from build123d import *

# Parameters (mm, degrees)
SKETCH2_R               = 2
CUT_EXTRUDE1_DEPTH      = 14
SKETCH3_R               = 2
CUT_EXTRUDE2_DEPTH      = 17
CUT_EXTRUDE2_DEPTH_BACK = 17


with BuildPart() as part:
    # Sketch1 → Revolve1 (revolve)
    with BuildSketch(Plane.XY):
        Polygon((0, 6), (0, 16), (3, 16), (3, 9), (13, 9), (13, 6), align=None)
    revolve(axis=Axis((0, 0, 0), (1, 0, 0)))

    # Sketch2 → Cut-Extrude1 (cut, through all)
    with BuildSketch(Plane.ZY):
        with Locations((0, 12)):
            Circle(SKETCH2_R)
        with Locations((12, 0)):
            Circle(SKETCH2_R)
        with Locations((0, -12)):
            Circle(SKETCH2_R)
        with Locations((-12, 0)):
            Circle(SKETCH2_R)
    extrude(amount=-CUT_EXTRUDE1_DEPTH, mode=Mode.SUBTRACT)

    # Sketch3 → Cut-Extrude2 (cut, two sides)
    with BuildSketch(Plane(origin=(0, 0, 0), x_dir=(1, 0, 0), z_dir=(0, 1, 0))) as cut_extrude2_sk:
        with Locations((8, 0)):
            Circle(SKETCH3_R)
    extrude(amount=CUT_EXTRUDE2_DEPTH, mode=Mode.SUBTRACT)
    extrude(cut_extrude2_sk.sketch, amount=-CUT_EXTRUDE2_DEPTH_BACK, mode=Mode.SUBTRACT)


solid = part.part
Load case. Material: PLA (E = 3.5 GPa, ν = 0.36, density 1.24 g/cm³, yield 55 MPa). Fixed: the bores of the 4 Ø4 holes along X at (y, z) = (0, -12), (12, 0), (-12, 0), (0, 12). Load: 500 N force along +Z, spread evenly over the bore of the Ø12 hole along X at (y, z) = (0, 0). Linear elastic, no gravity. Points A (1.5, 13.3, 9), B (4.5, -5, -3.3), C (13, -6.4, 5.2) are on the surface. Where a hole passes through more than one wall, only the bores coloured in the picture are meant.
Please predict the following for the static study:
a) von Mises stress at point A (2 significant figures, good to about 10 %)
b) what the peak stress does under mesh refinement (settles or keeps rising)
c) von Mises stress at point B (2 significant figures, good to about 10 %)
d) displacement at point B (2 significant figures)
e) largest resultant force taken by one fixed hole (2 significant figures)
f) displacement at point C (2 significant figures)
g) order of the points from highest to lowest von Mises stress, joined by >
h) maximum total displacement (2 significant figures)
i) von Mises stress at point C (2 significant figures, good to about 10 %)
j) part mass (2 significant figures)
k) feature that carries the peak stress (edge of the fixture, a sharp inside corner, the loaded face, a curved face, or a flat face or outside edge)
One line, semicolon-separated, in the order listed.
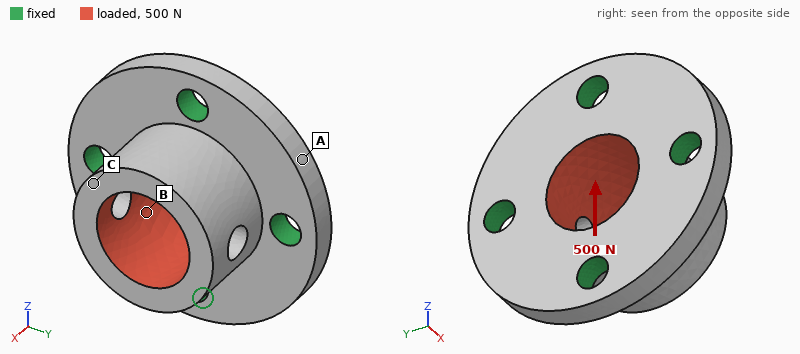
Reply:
1.5 MPa; keeps rising; 5.2 MPa; 17 µm; 180 N; 51 µm; B > C > A; 58 µm; 2.9 MPa; 4.0 g; edge of the fixture
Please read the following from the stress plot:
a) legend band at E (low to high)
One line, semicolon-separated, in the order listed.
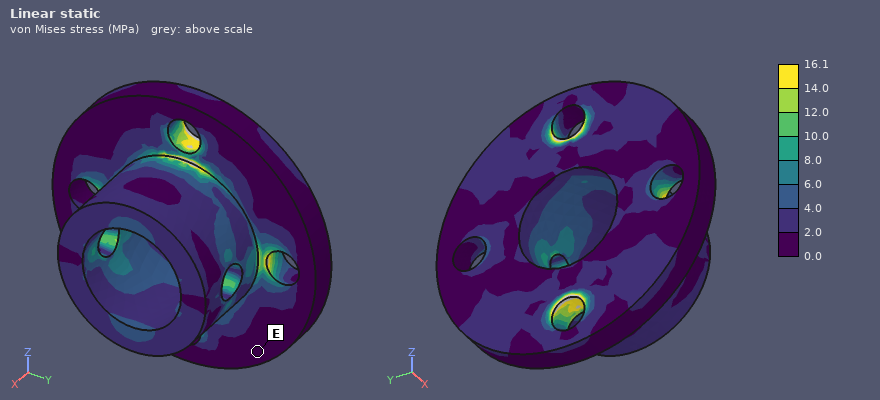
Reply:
0.0 to 2.0 MPa
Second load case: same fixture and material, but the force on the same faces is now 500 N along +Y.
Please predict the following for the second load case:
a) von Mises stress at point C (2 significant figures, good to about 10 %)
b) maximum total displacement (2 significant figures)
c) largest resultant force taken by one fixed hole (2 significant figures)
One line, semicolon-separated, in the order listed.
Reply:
3.4 MPa; 53 µm; 180 N
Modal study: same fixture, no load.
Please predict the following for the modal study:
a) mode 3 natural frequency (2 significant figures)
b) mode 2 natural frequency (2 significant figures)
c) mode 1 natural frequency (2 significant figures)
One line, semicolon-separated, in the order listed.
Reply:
13 kHz; 12 kHz; 11 kHz
